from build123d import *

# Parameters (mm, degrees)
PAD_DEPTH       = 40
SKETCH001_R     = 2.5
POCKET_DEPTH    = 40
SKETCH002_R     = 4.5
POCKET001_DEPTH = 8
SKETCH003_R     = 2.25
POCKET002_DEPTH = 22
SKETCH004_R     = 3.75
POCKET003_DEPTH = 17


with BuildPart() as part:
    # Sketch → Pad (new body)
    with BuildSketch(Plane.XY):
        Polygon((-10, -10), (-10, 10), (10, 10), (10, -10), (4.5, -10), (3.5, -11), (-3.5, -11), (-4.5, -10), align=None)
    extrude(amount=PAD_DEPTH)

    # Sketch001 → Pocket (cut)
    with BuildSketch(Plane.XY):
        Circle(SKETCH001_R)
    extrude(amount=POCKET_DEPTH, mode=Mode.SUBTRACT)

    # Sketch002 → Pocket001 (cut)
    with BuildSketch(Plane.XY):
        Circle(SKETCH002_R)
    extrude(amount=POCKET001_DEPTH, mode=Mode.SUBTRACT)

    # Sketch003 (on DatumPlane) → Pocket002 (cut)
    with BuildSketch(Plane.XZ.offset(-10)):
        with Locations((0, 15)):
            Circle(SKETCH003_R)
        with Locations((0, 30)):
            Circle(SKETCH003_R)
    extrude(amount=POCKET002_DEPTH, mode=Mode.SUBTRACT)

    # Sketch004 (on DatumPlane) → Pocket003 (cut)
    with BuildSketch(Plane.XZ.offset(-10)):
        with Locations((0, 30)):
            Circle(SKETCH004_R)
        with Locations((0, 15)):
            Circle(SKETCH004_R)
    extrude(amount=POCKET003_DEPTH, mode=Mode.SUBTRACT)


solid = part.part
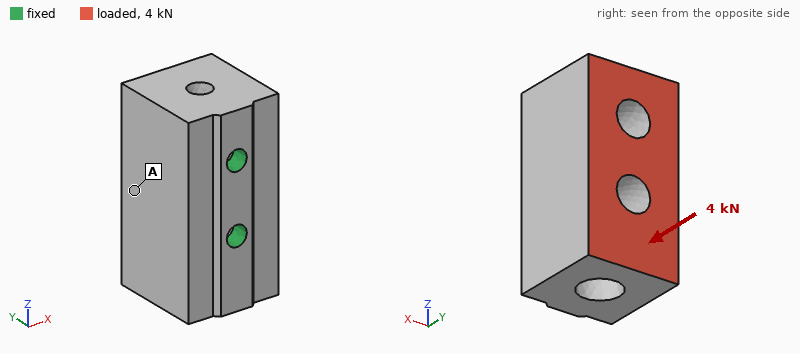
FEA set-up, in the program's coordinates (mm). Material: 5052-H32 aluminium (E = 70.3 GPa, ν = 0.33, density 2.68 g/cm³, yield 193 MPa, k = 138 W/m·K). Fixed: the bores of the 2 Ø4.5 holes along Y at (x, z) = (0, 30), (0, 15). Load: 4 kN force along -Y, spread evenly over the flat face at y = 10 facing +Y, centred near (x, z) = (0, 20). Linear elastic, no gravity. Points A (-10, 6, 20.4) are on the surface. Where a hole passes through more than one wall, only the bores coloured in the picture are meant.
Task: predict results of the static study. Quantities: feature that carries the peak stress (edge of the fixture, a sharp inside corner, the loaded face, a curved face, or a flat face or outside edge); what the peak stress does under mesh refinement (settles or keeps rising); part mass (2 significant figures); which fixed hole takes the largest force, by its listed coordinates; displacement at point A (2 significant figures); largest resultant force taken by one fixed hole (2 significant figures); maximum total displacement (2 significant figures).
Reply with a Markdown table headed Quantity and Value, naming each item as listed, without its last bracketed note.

| Quantity | Value |
|---|---|
| feature that carries the peak stress | edge of the fixture |
| what the peak stress does under mesh refinement | keeps rising |
| part mass | 37 g |
| which fixed hole takes the largest force, by its listed coordinates | (0, 15) |
| displacement at point A | 6.2 µm |
| largest resultant force taken by one fixed hole | 2.6 kN |
| maximum total displacement | 15 µm |
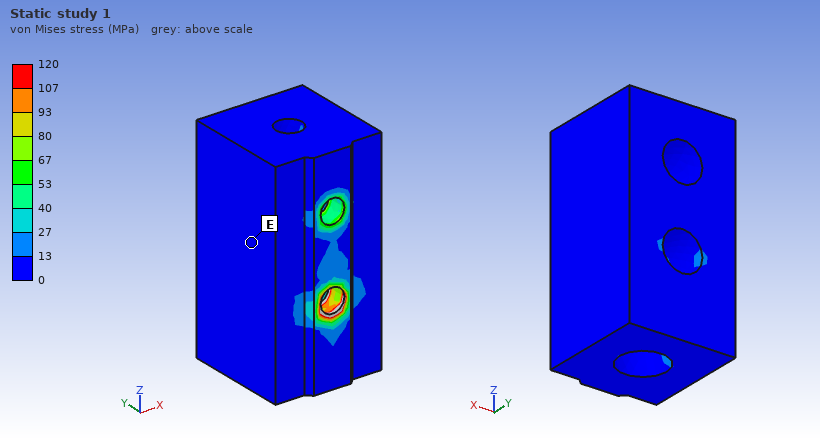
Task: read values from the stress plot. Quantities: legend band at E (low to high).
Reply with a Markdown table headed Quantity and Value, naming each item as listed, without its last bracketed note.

| Quantity | Value |
|---|---|
| legend band at E | 0 to 13 MPa |
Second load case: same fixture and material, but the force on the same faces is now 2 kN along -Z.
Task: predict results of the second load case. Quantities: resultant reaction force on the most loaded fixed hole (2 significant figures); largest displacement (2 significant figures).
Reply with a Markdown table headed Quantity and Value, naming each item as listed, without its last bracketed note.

| Quantity | Value |
|---|---|
| resultant reaction force on the most loaded fixed hole | 2.3 kN |
| largest displacement | 26 µm |
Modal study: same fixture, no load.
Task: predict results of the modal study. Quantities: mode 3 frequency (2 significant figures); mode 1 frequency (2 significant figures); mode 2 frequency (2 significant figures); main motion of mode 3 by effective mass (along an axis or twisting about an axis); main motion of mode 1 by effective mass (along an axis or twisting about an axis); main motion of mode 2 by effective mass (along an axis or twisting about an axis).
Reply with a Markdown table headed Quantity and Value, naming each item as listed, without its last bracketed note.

| Quantity | Value |
|---|---|
| mode 3 frequency | 15 kHz |
| mode 1 frequency | 6500 Hz |
| mode 2 frequency | 12 kHz |
| main motion of mode 3 by effective mass | twisting about Y |
| main motion of mode 1 by effective mass | along X |
| main motion of mode 2 by effective mass | along Z |
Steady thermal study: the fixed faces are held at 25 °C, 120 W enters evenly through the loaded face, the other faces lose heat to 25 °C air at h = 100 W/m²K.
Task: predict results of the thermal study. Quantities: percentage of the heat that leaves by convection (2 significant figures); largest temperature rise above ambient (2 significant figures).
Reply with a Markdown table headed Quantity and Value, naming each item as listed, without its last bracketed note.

| Quantity | Value |
|---|---|
| percentage of the heat that leaves by convection | 9.7 % |
| largest temperature rise above ambient | 45 K |
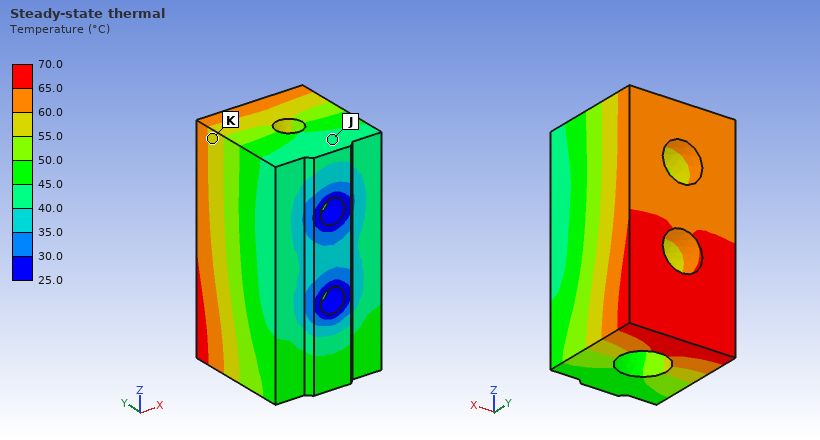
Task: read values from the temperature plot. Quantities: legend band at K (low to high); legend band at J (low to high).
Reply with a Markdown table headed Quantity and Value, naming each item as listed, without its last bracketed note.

| Quantity | Value |
|---|---|
| legend band at K | 55.0 to 60.0 °C |
| legend band at J | 40.0 to 45.0 °C |
